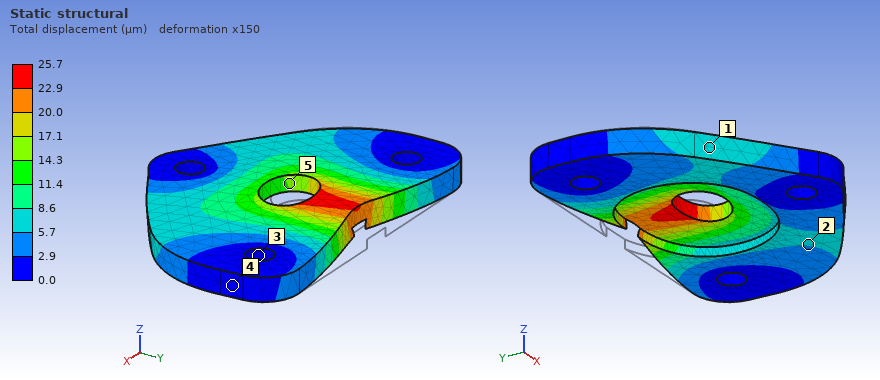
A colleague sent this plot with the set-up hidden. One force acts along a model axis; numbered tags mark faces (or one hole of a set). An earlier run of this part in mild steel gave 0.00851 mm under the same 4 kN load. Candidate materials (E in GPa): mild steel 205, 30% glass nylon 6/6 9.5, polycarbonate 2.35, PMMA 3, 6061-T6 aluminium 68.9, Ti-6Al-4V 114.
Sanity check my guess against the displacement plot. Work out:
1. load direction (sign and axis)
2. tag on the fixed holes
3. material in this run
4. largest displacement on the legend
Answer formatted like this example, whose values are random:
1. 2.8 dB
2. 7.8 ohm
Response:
1. -Y
2. 3
3. 6061-T6 aluminium
4. 25.7 µm
